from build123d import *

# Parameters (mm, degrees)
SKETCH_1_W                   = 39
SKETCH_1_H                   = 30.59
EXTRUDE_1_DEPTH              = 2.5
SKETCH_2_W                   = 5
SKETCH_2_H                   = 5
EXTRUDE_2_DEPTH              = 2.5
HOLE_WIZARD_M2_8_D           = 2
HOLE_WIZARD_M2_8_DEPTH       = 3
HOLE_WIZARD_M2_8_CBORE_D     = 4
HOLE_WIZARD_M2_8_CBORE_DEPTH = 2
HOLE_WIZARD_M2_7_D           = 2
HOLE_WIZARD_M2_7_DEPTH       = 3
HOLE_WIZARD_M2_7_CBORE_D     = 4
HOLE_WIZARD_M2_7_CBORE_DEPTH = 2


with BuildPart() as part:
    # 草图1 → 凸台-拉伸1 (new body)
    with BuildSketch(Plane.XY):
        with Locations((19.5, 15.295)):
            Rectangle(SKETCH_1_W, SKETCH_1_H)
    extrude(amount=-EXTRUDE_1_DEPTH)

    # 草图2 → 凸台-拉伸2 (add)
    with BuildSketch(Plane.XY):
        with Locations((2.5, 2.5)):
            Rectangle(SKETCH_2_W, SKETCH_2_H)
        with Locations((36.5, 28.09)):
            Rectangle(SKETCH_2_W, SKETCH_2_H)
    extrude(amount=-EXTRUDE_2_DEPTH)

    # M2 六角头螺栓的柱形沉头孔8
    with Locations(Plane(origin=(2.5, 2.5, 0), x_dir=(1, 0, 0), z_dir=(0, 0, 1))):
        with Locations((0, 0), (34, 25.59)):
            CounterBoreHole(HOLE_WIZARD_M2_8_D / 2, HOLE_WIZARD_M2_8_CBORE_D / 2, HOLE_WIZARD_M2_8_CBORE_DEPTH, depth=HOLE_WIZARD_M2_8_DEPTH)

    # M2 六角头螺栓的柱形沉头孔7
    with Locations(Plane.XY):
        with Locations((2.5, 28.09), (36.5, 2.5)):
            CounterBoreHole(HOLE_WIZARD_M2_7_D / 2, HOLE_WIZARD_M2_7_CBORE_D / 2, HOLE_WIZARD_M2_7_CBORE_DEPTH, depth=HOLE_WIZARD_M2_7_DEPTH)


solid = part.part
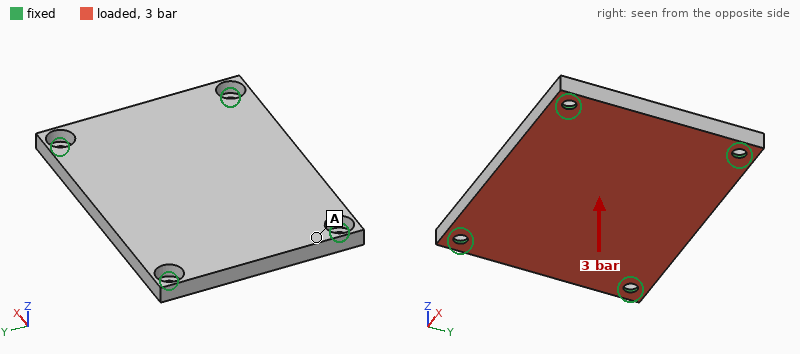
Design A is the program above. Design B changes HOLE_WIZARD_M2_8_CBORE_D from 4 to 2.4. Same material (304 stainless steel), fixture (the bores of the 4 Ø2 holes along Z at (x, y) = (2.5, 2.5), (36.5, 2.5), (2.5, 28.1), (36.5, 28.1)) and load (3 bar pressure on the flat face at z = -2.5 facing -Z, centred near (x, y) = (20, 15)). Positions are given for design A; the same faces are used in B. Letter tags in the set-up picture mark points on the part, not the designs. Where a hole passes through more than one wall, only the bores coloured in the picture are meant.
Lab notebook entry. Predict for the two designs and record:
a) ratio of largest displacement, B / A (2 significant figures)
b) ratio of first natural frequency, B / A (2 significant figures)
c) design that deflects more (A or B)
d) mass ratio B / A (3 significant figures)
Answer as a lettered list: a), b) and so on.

a) 0.91
b) 1.0
c) A
d) 1.01
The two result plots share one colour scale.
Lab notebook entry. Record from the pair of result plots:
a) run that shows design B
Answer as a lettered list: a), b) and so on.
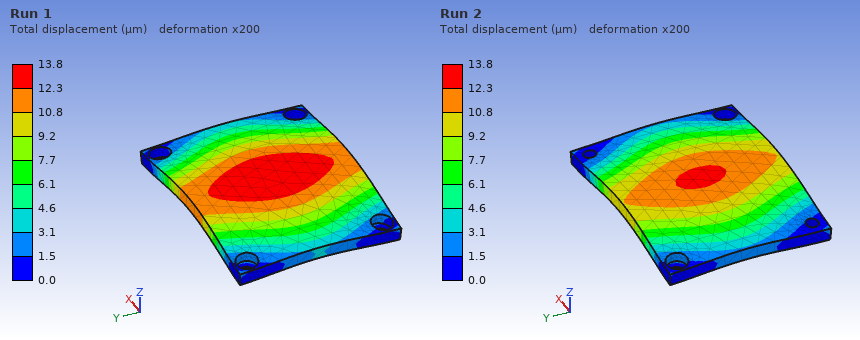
a) Run 2
